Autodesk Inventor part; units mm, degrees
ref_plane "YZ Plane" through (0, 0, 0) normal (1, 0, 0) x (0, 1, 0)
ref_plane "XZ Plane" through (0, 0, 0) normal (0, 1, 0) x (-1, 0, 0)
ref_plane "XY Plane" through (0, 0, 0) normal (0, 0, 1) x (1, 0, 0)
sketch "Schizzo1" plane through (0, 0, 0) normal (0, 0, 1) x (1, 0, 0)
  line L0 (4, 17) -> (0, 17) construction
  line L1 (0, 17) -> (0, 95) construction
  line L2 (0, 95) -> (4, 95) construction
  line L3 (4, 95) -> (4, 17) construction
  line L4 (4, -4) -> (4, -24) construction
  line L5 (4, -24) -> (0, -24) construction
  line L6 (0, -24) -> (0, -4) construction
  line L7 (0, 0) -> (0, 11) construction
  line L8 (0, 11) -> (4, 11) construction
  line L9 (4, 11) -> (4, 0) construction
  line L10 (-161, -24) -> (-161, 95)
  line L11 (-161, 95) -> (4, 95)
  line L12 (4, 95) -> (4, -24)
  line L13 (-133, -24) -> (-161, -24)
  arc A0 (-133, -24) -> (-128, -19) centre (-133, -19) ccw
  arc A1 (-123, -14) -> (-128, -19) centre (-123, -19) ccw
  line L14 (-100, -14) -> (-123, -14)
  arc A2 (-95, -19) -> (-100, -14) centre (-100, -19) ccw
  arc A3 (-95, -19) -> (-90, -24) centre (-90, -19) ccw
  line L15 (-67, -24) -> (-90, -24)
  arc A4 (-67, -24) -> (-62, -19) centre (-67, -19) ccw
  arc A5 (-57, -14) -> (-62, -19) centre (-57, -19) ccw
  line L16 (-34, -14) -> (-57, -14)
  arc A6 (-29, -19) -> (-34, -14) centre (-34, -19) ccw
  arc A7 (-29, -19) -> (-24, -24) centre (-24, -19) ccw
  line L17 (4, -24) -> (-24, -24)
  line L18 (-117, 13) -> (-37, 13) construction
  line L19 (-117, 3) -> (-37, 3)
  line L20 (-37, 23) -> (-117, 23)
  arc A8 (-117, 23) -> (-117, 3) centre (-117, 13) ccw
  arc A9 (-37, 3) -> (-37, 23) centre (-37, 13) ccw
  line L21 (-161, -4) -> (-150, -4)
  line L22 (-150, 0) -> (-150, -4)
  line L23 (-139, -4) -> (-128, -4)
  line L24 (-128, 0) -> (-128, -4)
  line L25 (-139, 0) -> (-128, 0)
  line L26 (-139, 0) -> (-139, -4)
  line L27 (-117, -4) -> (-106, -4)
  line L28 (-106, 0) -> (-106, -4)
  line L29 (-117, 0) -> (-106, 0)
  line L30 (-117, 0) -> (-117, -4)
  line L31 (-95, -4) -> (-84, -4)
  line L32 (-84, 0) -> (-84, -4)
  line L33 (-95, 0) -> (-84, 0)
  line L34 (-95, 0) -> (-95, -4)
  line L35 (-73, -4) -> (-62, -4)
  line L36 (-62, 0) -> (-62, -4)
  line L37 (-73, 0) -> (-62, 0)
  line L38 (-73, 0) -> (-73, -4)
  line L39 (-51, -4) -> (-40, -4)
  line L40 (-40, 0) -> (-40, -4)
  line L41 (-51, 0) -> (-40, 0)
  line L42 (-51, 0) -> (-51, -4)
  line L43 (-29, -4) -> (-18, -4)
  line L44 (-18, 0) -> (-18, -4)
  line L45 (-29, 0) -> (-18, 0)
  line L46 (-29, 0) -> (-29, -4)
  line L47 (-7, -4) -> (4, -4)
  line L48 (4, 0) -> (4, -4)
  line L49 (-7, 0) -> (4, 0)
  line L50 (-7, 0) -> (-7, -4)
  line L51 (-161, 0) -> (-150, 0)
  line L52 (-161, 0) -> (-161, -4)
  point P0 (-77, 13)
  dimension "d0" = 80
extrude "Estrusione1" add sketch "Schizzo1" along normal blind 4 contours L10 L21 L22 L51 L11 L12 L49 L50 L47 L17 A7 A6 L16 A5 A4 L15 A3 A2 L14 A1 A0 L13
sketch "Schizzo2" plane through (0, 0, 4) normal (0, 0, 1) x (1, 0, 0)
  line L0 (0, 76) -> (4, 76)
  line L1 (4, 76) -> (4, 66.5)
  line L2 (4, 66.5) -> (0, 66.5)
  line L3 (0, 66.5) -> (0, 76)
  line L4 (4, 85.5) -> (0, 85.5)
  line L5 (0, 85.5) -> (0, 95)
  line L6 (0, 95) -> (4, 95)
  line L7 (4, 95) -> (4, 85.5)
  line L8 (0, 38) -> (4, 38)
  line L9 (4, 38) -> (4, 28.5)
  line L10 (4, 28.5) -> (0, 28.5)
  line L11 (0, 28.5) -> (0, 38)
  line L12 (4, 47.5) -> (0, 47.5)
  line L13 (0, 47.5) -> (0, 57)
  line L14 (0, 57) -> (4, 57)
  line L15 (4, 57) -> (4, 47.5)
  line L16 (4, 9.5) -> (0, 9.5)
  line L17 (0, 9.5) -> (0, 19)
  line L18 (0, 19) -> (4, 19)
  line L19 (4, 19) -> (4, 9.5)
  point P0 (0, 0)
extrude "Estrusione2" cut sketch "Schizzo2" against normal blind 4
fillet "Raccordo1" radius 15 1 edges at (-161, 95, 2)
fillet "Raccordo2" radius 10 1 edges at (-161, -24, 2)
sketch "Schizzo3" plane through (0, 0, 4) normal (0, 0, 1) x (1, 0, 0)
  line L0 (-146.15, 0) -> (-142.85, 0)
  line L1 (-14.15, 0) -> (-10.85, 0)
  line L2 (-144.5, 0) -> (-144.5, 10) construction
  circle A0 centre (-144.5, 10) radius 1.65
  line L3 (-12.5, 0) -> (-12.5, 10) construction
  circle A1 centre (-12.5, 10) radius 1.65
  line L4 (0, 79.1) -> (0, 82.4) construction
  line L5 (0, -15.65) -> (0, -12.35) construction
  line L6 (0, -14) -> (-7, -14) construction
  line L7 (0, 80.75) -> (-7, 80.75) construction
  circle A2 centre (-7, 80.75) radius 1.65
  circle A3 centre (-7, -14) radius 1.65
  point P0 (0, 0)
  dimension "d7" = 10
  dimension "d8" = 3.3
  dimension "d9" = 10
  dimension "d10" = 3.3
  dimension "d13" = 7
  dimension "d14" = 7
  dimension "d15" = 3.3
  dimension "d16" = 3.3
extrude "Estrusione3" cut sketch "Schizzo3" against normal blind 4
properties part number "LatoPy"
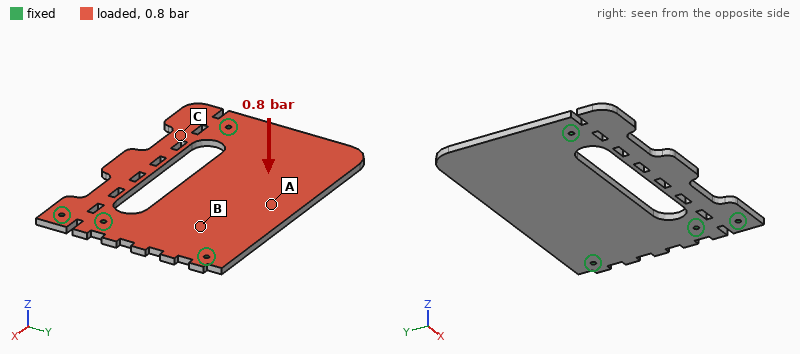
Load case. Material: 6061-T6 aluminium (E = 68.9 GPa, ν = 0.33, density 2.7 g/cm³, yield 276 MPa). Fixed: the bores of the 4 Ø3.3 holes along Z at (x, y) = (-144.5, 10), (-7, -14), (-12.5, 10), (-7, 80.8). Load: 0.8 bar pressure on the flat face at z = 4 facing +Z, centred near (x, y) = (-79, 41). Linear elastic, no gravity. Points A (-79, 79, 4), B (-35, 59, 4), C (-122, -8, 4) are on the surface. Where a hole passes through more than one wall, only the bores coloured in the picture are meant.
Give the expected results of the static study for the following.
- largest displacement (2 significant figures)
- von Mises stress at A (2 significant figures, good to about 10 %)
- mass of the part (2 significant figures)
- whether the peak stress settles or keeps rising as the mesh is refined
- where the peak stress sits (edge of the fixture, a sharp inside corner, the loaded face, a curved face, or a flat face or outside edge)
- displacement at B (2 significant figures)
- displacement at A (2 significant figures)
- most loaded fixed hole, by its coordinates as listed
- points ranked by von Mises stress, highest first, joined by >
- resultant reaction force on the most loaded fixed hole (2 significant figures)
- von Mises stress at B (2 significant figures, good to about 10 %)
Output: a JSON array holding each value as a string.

["1.5 mm", "43 MPa", "180 g", "keeps rising", "edge of the fixture", "0.24 mm", "0.86 mm", "(-144.5, 10)", "A > B > C", "610 N", "32 MPa"]
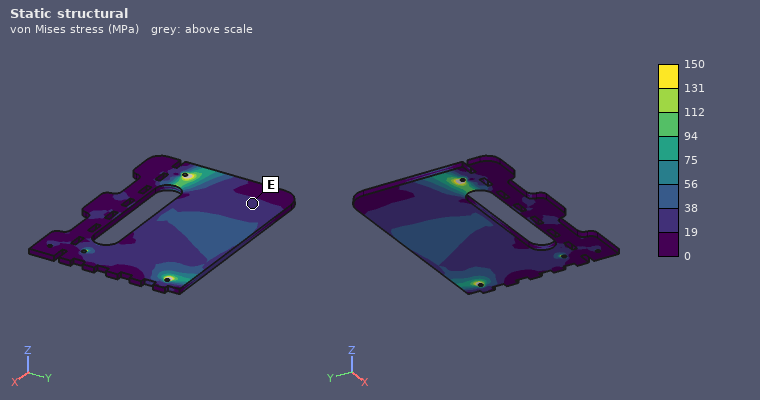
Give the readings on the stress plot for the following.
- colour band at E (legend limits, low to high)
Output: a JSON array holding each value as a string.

["19 to 38 MPa"]
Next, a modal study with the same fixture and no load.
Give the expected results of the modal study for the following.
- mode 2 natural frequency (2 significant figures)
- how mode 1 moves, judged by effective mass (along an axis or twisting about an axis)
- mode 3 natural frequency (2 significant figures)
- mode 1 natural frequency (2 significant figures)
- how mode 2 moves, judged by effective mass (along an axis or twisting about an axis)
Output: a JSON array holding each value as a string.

["1000 Hz", "along Z", "1100 Hz", "470 Hz", "along Z"]
